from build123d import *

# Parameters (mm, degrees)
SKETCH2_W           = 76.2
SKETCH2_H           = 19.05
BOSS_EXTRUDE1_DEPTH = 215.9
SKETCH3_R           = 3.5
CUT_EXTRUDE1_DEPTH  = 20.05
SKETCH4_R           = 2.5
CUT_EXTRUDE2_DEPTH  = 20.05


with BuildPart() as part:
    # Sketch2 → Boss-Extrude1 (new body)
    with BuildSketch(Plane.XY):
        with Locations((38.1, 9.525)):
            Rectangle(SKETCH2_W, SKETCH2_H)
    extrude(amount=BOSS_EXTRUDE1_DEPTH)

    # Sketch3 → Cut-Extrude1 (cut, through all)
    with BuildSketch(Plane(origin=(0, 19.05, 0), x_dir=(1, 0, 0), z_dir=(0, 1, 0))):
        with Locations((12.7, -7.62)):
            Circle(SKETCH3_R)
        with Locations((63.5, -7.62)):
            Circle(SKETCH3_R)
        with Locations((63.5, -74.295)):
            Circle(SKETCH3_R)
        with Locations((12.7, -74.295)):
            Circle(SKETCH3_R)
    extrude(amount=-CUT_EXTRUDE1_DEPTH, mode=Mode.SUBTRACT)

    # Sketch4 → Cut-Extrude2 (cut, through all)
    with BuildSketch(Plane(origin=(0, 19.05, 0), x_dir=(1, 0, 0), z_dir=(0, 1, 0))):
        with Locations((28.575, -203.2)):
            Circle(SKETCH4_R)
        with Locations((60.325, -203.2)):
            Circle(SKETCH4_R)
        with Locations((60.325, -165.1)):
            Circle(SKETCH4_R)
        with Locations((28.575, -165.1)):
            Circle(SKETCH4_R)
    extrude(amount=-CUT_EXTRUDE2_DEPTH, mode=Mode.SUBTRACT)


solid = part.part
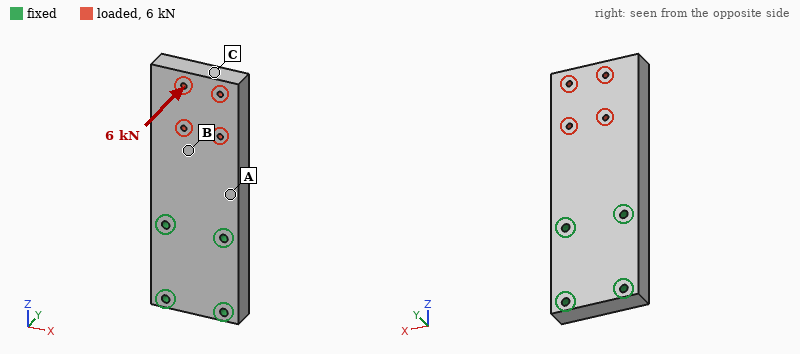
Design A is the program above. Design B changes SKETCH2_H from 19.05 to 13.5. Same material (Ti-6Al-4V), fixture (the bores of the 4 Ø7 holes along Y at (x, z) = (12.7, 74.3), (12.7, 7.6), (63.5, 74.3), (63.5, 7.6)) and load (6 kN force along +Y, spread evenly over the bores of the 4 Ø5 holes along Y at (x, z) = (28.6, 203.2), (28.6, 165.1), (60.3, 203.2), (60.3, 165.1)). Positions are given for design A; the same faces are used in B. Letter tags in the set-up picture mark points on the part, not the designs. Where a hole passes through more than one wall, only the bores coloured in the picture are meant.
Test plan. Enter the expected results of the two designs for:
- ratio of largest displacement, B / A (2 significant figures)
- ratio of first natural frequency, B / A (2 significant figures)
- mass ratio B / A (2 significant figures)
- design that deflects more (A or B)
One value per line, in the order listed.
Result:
2.7
0.72
0.71
B
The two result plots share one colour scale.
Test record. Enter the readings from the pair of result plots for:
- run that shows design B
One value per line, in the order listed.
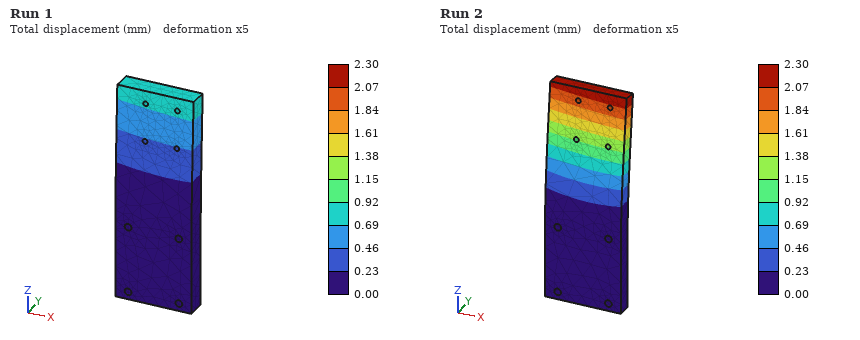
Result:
Run 2
